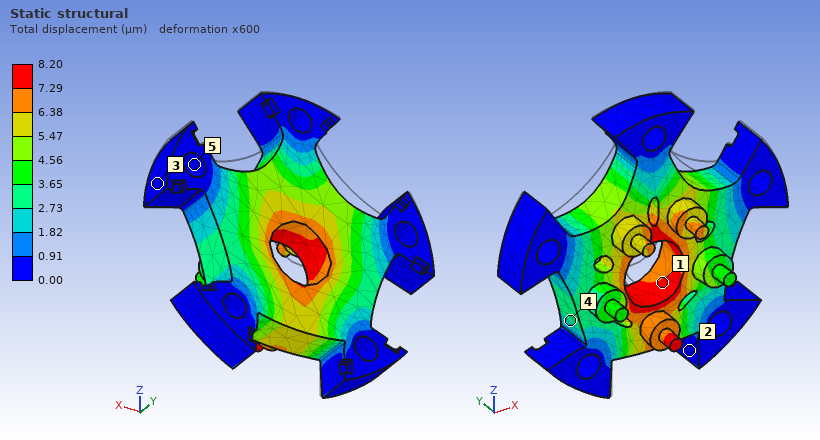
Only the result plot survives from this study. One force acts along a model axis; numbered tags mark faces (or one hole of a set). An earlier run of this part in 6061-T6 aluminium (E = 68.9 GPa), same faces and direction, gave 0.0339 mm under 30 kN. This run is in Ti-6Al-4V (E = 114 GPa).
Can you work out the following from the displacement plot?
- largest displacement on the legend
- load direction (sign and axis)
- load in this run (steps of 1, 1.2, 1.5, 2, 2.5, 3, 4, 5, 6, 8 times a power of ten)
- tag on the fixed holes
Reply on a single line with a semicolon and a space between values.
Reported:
8.20 µm; -Z; 12 kN; 5
